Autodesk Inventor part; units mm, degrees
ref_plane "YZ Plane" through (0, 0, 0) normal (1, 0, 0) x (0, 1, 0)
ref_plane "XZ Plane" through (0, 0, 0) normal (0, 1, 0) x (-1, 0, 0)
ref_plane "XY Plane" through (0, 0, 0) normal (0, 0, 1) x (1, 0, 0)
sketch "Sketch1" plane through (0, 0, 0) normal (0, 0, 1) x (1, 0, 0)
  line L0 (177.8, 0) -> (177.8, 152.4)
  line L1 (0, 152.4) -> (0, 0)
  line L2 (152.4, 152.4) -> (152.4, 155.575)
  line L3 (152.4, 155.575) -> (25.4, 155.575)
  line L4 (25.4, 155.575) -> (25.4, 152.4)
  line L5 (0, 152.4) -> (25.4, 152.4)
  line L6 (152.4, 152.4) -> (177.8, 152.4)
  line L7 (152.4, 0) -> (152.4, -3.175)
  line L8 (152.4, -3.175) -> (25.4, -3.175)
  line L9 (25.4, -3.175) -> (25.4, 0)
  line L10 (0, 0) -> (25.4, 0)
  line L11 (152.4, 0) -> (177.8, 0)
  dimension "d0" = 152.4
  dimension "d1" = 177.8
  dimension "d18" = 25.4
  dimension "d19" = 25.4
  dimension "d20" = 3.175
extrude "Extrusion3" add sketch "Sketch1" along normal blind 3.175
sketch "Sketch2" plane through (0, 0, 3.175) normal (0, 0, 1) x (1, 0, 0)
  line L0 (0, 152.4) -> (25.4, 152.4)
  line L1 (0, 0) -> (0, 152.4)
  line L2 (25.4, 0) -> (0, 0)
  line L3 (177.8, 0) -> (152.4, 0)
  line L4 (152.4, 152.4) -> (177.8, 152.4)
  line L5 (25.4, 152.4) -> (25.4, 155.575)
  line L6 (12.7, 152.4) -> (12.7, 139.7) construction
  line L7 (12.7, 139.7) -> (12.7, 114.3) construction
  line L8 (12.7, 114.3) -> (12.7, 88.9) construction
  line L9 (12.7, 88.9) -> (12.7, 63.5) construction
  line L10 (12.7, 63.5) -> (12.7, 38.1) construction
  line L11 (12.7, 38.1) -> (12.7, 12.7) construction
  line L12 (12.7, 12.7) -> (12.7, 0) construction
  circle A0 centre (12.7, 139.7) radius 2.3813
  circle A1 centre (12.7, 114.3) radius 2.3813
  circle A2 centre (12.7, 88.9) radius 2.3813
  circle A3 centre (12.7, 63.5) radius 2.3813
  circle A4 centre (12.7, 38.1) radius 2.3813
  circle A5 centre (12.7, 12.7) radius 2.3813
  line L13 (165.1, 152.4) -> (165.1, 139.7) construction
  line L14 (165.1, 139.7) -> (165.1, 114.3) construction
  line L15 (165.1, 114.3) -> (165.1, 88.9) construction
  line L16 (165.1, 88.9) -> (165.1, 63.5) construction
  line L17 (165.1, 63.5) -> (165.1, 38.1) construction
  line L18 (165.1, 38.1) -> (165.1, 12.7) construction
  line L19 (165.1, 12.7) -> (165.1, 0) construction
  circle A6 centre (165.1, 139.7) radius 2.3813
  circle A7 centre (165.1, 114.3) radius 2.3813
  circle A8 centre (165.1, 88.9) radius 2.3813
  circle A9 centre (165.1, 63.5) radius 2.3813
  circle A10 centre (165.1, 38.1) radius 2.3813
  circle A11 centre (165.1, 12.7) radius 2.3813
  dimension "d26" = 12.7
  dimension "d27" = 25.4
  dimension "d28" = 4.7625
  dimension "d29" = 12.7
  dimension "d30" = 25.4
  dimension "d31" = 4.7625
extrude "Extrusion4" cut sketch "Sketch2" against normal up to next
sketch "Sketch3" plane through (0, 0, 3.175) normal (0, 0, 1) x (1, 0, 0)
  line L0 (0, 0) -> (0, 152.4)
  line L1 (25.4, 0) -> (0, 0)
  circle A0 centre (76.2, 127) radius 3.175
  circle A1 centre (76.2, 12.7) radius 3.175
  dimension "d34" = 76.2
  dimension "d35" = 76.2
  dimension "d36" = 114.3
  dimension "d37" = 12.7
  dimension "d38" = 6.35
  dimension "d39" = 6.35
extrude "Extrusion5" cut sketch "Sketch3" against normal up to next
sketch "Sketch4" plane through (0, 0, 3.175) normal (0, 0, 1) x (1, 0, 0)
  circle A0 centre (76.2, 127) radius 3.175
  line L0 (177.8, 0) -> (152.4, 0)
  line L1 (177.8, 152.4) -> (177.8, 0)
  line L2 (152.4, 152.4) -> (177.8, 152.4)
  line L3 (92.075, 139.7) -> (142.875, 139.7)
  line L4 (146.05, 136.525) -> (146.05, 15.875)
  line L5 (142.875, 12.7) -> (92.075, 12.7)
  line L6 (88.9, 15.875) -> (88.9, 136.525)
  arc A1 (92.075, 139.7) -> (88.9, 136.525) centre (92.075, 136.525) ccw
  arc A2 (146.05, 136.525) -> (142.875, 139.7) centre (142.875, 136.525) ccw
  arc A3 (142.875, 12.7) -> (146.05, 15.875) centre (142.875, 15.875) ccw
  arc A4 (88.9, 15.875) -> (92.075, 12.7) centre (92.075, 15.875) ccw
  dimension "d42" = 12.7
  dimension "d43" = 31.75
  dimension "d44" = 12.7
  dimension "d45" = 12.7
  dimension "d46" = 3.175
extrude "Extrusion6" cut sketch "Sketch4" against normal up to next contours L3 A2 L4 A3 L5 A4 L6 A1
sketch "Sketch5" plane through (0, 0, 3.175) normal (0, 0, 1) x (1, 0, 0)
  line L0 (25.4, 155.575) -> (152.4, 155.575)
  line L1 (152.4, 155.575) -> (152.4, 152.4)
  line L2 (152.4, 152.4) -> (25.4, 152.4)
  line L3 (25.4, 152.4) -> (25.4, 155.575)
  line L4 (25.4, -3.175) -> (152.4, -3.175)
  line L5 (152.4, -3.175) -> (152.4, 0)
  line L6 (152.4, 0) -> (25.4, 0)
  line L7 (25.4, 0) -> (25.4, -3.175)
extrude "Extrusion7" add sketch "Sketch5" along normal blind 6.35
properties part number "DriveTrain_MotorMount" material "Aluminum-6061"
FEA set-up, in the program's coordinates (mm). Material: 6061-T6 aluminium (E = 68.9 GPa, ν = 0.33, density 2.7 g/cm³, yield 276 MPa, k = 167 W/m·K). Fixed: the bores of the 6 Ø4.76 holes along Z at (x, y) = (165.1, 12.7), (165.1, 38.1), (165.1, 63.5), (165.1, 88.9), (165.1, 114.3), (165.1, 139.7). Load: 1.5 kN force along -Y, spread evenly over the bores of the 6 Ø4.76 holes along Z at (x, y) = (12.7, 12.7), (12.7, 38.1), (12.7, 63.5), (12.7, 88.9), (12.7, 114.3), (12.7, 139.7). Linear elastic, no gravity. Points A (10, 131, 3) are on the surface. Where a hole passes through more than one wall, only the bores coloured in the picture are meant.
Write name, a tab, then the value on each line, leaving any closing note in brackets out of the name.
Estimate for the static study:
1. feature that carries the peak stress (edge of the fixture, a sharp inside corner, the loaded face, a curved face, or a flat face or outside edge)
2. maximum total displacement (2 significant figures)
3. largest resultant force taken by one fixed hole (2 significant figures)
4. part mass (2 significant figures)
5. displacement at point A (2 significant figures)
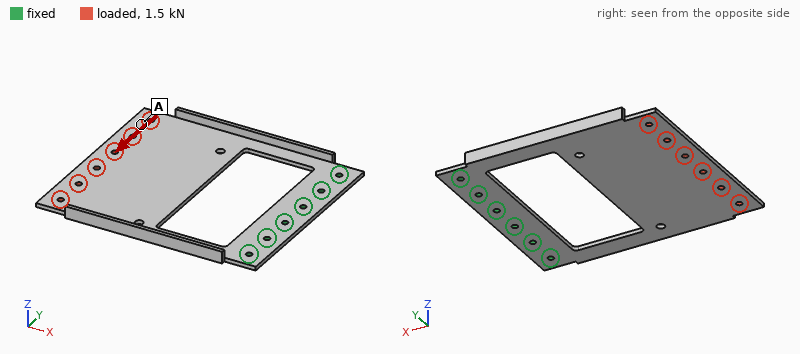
feature that carries the peak stress	a curved face
maximum total displacement	0.55 mm
largest resultant force taken by one fixed hole	2.3 kN
part mass	190 g
displacement at point A	0.52 mm
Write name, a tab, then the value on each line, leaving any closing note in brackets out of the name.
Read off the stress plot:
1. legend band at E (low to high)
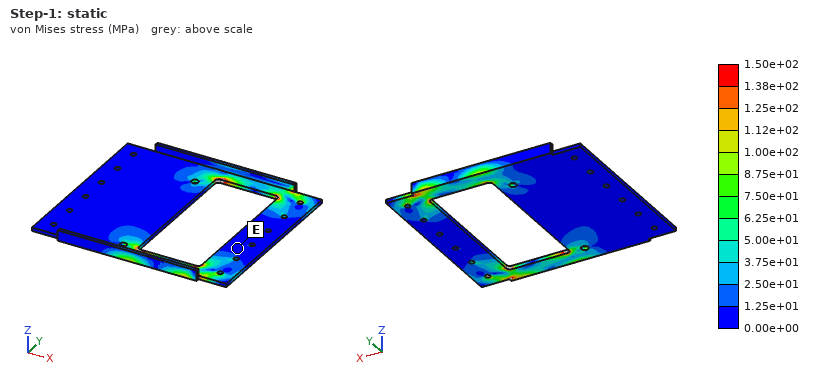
legend band at E	0.00e+00 to 1.25e+01 MPa
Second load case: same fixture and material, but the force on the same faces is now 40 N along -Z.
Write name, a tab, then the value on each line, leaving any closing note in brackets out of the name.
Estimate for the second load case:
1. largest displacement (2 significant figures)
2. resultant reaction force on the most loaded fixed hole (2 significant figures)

largest displacement	2.8 mm
resultant reaction force on the most loaded fixed hole	63 N
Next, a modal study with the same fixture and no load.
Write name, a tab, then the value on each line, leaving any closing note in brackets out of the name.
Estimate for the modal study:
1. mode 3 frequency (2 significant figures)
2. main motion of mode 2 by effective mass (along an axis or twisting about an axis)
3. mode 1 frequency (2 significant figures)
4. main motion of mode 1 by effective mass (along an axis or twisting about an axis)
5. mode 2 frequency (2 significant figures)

mode 3 frequency	610 Hz
main motion of mode 2 by effective mass	twisting about X
mode 1 frequency	74 Hz
main motion of mode 1 by effective mass	along Z
mode 2 frequency	200 Hz
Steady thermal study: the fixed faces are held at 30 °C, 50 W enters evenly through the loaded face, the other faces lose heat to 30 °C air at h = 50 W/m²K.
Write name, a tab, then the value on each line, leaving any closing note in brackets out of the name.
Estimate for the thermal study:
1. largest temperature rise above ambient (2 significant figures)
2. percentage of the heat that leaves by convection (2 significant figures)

largest temperature rise above ambient	43 K
percentage of the heat that leaves by convection	93 %
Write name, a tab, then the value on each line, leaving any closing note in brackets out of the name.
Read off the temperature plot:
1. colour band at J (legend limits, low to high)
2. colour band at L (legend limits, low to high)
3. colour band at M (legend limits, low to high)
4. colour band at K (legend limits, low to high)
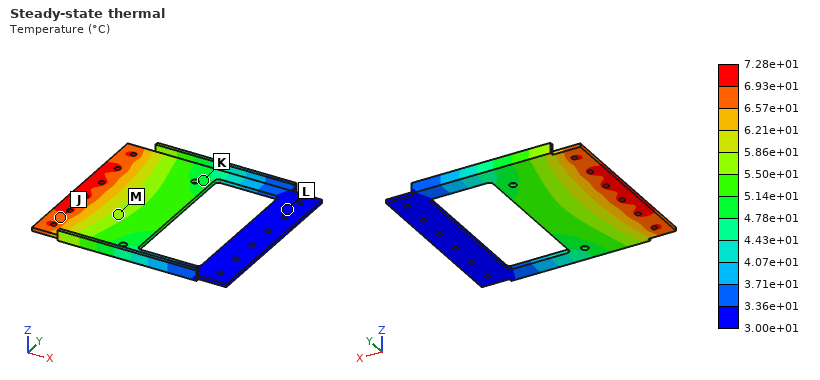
colour band at J	6.57e+01 to 6.93e+01 °C
colour band at L	3.00e+01 to 3.36e+01 °C
colour band at M	5.50e+01 to 5.86e+01 °C
colour band at K	4.78e+01 to 5.14e+01 °C
